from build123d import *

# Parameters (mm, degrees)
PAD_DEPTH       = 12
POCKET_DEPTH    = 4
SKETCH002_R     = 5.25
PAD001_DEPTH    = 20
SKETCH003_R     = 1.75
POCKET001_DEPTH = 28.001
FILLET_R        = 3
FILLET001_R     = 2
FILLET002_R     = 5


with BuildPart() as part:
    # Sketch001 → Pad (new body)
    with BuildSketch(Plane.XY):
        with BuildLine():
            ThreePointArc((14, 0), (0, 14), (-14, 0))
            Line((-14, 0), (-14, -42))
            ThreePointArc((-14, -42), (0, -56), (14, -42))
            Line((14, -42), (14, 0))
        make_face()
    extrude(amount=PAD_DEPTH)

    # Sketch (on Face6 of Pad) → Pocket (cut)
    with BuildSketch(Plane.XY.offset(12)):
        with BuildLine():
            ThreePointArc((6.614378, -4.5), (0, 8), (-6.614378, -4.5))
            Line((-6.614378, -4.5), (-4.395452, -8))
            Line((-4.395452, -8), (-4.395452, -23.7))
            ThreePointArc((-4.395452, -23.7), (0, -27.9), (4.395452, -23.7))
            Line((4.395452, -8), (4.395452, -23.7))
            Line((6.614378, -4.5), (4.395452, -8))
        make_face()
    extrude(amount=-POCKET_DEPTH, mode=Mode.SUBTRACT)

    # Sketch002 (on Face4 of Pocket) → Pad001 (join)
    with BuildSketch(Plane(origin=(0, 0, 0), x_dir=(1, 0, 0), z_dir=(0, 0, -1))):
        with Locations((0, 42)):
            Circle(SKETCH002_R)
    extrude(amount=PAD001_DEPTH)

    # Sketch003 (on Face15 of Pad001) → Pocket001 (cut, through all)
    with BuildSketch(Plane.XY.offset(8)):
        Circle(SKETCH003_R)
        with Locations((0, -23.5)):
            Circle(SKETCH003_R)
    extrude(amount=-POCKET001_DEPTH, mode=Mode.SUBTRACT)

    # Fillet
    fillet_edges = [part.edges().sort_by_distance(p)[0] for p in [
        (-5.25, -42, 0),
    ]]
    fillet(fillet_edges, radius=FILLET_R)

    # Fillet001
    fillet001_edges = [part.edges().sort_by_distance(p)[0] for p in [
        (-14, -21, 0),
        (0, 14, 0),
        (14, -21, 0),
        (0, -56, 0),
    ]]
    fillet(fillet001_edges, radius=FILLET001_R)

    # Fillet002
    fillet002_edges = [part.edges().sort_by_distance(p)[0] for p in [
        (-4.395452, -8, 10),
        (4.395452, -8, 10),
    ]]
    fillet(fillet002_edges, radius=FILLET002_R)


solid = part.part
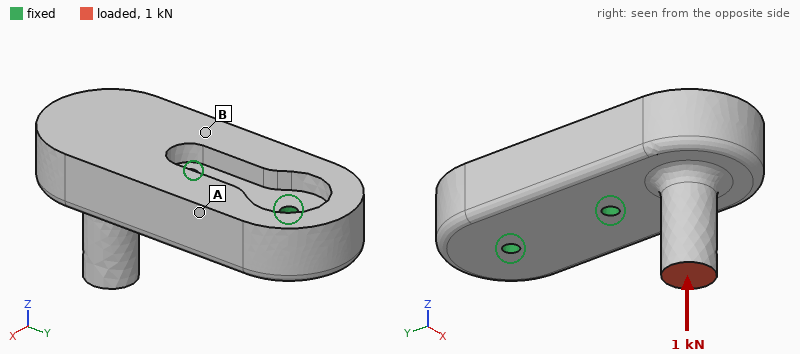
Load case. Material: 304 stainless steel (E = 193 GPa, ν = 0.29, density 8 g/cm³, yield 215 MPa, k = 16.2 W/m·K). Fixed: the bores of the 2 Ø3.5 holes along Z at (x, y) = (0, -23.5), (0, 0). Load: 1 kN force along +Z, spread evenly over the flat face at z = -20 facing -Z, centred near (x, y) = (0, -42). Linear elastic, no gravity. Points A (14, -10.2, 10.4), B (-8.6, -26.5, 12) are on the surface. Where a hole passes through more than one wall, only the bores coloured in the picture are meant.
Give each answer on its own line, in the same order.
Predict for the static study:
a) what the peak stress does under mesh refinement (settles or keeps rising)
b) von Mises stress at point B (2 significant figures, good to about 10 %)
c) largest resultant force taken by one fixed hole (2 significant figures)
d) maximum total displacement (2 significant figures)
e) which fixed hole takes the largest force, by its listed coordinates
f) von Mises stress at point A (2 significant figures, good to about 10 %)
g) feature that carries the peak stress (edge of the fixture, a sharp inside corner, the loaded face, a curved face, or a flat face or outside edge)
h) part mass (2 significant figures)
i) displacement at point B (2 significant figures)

keeps rising
23 MPa
1.5 kN
16 µm
(0, -23.5)
7.4 MPa
edge of the fixture
170 g
2.4 µm
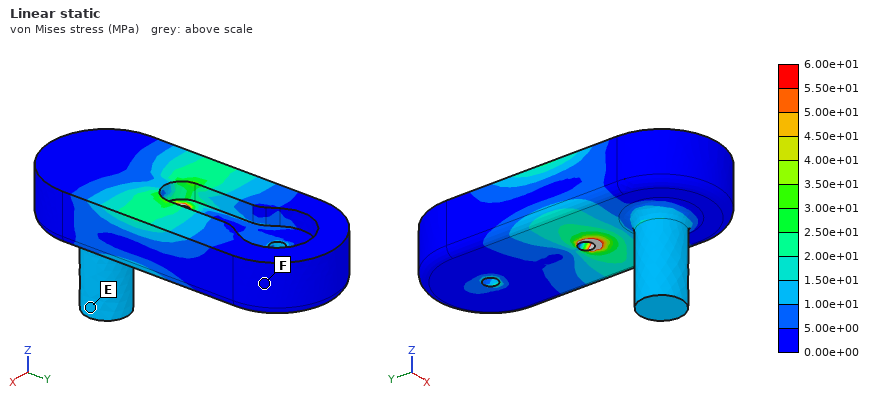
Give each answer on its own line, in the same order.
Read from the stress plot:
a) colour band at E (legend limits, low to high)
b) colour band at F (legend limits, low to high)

1.00e+01 to 1.50e+01 MPa
0.00e+00 to 5.00e+00 MPa
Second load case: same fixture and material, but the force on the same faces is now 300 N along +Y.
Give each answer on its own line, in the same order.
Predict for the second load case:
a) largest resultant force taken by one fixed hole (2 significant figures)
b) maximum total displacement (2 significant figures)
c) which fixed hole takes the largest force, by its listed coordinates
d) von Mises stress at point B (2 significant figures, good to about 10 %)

420 N
17 µm
(0, -23.5)
11 MPa
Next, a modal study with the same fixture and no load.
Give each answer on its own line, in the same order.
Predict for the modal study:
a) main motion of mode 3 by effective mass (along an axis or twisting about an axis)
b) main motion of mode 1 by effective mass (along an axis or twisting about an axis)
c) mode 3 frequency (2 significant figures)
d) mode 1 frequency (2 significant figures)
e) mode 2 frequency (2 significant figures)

along X
along Z
9900 Hz
5700 Hz
8000 Hz
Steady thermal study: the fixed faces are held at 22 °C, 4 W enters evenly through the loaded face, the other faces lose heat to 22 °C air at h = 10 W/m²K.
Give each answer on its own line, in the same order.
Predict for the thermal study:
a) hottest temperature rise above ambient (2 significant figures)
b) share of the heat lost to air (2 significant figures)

73 K
16 %
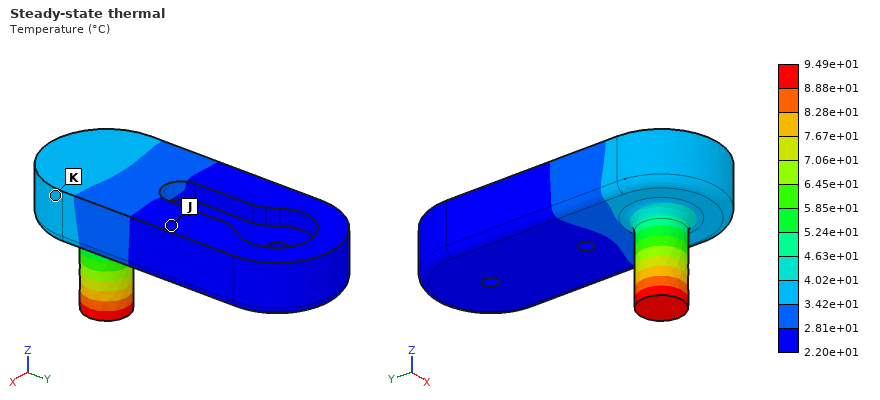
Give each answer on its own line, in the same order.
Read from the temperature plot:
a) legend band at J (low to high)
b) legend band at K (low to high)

2.20e+01 to 2.81e+01 °C
3.42e+01 to 4.02e+01 °C
